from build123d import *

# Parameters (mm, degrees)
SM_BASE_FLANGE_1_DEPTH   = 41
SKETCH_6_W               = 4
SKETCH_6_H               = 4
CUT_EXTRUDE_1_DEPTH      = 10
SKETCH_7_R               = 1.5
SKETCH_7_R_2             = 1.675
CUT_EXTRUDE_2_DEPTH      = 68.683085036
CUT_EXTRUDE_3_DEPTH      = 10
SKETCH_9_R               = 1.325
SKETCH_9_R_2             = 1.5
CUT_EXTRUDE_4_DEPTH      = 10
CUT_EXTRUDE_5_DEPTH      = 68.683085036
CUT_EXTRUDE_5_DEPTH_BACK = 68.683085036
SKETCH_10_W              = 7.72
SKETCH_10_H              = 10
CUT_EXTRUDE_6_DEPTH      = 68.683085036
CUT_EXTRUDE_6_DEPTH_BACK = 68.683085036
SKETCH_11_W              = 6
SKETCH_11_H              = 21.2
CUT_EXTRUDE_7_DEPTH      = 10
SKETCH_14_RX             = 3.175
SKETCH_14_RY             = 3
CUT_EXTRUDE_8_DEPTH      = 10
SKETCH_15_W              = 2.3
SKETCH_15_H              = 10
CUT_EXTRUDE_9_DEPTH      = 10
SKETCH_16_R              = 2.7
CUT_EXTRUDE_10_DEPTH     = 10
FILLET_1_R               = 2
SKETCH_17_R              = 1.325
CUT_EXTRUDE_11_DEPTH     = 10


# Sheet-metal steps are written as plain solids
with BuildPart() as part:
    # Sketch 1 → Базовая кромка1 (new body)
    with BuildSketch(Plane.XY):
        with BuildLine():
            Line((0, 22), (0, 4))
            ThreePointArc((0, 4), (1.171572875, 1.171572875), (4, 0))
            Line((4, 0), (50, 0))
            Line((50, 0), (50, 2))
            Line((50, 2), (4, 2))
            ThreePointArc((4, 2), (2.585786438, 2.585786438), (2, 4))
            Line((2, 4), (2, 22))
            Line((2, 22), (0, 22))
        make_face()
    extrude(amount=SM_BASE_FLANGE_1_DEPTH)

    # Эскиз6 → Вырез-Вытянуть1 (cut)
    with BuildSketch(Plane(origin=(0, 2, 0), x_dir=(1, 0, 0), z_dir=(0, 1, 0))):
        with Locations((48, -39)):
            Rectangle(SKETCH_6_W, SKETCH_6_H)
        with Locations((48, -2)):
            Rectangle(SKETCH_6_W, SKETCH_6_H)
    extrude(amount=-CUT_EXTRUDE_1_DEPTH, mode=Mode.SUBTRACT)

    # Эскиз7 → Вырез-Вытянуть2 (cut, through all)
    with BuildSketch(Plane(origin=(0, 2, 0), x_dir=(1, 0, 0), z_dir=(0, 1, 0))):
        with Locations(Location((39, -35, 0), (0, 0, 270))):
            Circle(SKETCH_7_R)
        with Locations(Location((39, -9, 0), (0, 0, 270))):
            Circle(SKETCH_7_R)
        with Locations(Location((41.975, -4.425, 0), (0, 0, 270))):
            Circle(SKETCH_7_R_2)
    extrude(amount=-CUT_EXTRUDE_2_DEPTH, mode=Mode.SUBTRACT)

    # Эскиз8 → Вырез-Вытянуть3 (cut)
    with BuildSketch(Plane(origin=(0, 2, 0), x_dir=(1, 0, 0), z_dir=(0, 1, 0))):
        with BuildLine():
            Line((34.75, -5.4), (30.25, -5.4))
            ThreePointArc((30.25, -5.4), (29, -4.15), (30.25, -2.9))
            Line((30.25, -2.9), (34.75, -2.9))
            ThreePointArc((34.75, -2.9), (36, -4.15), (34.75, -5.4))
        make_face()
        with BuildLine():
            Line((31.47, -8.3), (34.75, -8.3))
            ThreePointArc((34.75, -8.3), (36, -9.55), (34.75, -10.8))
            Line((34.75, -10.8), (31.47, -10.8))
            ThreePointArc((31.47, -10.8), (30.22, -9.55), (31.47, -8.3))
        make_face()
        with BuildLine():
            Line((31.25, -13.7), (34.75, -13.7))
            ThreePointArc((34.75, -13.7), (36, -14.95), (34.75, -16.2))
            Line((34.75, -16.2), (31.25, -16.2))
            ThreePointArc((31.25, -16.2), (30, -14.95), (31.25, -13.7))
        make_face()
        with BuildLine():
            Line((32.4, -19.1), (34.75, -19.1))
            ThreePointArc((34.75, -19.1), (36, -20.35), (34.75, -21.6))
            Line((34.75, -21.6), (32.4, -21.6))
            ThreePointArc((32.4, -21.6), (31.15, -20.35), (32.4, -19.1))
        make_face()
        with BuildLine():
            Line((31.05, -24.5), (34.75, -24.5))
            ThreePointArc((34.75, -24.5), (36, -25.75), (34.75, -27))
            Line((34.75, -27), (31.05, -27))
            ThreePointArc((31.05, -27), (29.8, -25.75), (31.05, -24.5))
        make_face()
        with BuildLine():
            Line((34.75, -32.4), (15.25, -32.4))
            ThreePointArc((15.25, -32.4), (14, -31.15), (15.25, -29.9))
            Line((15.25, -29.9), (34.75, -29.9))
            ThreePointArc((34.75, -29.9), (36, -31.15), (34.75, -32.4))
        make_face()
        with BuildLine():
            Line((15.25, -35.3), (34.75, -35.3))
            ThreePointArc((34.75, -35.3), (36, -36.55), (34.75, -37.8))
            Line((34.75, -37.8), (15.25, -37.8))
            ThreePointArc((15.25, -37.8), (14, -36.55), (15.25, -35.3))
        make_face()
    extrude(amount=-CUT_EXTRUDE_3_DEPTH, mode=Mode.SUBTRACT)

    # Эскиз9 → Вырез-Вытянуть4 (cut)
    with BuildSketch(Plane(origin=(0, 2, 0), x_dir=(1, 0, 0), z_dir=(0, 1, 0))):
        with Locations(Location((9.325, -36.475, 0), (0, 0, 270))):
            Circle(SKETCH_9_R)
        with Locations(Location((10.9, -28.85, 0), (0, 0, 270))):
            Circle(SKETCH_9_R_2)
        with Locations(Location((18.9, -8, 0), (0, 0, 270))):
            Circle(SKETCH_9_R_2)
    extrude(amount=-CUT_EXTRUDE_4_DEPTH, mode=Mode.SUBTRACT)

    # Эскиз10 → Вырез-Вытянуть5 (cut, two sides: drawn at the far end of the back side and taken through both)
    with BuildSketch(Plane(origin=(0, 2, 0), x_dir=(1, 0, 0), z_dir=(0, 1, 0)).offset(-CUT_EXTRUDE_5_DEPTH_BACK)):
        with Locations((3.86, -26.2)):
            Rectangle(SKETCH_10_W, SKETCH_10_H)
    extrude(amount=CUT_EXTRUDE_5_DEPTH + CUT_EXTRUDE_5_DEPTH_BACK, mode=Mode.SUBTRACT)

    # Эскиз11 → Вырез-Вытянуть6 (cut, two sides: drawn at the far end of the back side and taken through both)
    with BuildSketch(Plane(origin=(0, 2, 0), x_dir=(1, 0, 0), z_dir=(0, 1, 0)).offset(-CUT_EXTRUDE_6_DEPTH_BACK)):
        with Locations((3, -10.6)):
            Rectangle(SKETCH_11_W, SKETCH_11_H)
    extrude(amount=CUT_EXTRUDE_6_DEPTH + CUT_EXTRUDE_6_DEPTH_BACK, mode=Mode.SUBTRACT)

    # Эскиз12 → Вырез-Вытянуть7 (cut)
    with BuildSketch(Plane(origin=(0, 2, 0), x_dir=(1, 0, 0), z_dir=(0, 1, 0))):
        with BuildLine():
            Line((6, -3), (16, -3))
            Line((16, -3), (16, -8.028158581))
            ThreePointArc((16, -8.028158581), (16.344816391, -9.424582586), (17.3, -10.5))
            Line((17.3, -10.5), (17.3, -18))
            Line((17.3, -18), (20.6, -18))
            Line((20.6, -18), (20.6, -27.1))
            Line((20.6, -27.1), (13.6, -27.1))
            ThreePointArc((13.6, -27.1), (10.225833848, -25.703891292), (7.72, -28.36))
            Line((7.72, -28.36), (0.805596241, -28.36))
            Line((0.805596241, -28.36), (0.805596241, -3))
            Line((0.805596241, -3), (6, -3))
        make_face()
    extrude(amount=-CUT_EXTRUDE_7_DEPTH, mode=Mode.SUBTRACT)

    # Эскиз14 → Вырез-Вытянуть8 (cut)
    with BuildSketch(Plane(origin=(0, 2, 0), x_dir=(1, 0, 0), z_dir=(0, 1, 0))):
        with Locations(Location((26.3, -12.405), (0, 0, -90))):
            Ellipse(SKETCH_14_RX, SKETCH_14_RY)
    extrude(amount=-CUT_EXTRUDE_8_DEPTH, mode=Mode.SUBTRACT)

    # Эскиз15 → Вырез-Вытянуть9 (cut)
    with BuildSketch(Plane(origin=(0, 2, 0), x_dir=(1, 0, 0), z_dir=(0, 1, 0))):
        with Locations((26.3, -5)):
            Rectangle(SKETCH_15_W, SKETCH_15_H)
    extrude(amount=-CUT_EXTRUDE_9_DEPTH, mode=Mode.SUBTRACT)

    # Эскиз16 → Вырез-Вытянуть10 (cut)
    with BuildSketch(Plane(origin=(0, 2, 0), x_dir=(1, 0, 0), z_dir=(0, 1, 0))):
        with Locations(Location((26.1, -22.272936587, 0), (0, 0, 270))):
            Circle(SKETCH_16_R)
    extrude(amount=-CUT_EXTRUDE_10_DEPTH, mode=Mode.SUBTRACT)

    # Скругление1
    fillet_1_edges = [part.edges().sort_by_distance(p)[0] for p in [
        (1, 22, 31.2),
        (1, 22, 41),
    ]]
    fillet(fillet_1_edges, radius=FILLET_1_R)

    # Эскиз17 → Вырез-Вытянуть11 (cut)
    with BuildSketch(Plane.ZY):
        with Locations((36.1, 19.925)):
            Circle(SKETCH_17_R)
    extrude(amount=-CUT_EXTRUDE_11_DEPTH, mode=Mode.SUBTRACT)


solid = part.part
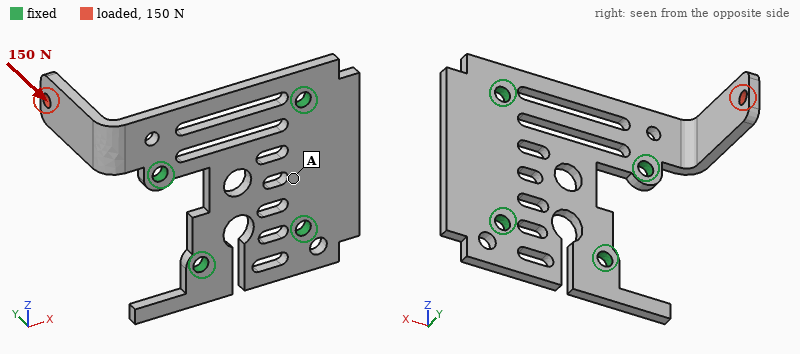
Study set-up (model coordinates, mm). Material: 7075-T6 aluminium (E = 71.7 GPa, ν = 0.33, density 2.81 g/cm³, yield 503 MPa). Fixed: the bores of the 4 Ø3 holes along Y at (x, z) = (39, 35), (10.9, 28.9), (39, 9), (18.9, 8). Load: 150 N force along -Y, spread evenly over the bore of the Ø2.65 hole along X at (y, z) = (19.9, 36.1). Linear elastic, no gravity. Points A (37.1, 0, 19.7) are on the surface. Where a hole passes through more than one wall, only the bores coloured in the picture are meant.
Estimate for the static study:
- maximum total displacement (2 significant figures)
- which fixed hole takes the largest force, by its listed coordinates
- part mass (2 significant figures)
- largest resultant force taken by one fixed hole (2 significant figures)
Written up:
0.62 mm
(10.9, 28.9)
8.0 g
170 N
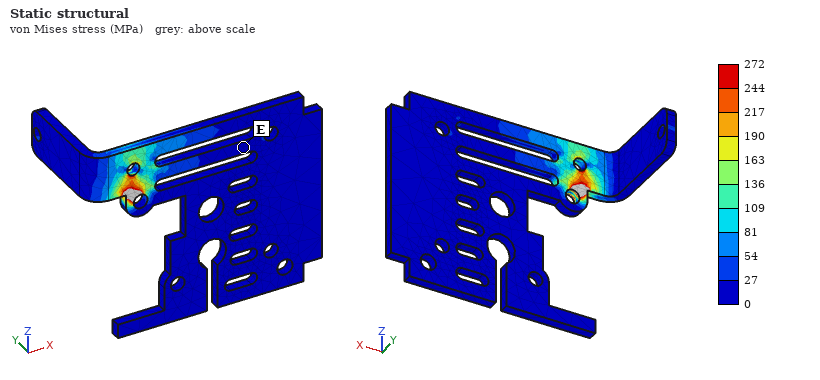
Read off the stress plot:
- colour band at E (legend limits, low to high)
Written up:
0 to 27 MPa
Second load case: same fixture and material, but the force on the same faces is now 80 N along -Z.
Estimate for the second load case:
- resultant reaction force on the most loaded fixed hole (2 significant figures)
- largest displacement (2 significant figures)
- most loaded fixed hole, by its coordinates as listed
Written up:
110 N
0.80 mm
(10.9, 28.9)
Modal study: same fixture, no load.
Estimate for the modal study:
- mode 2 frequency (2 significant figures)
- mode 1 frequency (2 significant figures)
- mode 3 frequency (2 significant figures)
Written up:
2500 Hz
2000 Hz
6800 Hz
